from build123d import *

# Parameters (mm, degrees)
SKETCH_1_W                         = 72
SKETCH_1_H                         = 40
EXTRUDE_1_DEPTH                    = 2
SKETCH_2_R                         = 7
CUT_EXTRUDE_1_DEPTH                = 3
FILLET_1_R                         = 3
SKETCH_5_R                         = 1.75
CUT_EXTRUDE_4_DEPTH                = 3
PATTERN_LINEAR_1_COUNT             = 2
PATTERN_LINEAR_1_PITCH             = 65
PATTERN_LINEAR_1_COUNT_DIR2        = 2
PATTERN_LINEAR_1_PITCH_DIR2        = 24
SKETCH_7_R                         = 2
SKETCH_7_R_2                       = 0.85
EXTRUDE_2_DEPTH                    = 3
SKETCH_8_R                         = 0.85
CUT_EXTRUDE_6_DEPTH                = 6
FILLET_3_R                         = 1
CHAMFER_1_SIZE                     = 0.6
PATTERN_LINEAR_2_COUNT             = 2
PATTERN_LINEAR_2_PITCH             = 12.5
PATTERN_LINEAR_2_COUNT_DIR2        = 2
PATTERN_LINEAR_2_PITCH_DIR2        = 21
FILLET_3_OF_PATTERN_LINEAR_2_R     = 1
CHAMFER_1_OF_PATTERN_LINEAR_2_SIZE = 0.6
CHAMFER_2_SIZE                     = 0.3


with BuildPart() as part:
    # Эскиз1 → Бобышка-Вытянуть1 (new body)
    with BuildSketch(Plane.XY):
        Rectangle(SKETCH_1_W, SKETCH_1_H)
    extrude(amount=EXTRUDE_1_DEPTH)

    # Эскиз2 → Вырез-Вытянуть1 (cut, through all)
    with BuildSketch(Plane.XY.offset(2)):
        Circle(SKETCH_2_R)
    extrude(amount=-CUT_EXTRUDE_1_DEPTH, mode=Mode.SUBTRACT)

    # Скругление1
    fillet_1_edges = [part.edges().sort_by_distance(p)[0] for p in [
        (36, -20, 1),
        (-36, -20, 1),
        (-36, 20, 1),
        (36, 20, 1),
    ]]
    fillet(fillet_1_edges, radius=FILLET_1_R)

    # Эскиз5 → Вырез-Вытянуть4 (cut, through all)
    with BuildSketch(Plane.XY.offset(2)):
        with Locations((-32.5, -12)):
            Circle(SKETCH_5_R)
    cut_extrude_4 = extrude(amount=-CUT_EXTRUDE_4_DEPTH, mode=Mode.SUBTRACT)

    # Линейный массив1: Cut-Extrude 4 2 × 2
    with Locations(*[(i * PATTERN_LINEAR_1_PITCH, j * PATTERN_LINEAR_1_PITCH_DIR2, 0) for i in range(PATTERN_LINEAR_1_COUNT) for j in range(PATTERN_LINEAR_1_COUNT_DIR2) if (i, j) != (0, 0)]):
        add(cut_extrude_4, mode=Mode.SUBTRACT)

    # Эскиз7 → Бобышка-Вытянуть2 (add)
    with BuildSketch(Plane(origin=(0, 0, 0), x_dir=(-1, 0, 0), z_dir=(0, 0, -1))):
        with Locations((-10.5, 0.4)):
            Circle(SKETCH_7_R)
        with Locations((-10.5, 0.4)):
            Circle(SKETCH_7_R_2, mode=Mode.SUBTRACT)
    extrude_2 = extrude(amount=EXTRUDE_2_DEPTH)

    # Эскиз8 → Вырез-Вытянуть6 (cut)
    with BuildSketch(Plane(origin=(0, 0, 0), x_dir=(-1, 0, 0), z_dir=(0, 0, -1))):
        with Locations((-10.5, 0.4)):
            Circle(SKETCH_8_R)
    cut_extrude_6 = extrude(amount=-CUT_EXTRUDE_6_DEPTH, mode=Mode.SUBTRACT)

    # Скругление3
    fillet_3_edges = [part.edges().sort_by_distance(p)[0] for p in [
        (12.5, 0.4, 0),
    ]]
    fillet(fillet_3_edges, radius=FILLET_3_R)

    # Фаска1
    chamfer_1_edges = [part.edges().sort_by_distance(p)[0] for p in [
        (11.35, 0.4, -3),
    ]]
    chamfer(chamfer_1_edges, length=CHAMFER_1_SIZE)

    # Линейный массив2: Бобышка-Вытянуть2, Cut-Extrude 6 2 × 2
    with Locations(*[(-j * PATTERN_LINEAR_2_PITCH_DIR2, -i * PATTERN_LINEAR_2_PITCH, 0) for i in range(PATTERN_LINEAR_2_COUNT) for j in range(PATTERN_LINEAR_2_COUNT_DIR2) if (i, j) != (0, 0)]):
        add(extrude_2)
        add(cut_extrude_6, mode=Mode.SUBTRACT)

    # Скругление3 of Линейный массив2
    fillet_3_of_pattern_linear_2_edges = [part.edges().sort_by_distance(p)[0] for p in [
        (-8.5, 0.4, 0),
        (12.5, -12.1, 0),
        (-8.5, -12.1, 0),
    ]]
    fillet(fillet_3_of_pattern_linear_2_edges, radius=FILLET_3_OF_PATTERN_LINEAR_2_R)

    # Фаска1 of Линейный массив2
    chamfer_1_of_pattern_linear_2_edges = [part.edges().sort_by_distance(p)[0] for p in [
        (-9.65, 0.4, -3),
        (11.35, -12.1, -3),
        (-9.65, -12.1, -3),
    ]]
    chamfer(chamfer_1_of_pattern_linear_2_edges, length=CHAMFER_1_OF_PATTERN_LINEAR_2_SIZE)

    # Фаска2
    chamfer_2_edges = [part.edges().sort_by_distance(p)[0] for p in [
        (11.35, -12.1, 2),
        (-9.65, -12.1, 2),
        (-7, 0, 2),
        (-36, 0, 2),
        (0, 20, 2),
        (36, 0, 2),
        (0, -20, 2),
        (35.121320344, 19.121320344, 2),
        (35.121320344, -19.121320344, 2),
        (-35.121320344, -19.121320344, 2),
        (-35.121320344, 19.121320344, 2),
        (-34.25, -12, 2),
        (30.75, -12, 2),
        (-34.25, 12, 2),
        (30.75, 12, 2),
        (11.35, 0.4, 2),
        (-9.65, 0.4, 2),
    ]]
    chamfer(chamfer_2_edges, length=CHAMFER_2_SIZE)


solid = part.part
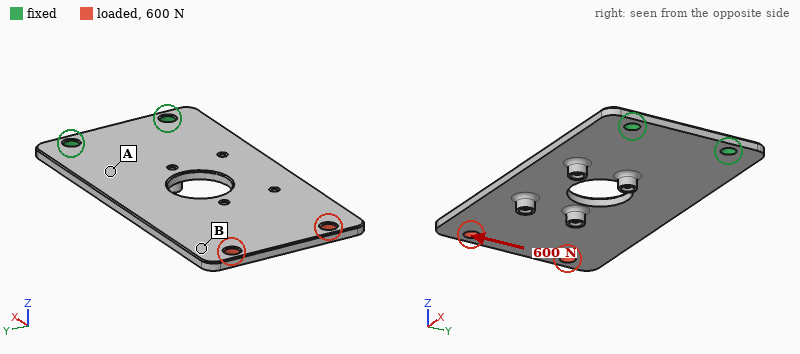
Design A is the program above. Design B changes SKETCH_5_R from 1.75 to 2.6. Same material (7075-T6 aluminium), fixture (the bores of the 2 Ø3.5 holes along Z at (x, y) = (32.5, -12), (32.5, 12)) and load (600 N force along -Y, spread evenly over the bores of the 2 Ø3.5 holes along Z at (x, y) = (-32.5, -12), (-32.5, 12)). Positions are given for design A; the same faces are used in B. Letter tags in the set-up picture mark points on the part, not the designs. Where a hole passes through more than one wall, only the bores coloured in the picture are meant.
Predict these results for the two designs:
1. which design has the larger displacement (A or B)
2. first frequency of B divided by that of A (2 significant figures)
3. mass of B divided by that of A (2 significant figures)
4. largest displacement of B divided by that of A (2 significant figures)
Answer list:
A
1.1
0.98
0.92
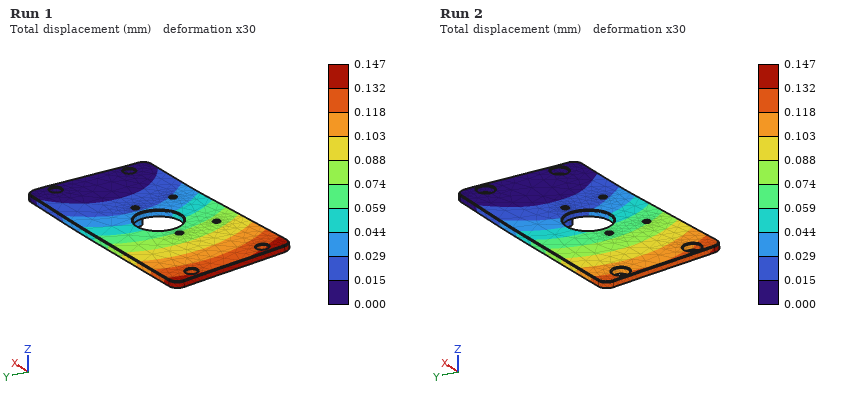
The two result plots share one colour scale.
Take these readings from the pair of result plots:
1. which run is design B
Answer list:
Run 2
